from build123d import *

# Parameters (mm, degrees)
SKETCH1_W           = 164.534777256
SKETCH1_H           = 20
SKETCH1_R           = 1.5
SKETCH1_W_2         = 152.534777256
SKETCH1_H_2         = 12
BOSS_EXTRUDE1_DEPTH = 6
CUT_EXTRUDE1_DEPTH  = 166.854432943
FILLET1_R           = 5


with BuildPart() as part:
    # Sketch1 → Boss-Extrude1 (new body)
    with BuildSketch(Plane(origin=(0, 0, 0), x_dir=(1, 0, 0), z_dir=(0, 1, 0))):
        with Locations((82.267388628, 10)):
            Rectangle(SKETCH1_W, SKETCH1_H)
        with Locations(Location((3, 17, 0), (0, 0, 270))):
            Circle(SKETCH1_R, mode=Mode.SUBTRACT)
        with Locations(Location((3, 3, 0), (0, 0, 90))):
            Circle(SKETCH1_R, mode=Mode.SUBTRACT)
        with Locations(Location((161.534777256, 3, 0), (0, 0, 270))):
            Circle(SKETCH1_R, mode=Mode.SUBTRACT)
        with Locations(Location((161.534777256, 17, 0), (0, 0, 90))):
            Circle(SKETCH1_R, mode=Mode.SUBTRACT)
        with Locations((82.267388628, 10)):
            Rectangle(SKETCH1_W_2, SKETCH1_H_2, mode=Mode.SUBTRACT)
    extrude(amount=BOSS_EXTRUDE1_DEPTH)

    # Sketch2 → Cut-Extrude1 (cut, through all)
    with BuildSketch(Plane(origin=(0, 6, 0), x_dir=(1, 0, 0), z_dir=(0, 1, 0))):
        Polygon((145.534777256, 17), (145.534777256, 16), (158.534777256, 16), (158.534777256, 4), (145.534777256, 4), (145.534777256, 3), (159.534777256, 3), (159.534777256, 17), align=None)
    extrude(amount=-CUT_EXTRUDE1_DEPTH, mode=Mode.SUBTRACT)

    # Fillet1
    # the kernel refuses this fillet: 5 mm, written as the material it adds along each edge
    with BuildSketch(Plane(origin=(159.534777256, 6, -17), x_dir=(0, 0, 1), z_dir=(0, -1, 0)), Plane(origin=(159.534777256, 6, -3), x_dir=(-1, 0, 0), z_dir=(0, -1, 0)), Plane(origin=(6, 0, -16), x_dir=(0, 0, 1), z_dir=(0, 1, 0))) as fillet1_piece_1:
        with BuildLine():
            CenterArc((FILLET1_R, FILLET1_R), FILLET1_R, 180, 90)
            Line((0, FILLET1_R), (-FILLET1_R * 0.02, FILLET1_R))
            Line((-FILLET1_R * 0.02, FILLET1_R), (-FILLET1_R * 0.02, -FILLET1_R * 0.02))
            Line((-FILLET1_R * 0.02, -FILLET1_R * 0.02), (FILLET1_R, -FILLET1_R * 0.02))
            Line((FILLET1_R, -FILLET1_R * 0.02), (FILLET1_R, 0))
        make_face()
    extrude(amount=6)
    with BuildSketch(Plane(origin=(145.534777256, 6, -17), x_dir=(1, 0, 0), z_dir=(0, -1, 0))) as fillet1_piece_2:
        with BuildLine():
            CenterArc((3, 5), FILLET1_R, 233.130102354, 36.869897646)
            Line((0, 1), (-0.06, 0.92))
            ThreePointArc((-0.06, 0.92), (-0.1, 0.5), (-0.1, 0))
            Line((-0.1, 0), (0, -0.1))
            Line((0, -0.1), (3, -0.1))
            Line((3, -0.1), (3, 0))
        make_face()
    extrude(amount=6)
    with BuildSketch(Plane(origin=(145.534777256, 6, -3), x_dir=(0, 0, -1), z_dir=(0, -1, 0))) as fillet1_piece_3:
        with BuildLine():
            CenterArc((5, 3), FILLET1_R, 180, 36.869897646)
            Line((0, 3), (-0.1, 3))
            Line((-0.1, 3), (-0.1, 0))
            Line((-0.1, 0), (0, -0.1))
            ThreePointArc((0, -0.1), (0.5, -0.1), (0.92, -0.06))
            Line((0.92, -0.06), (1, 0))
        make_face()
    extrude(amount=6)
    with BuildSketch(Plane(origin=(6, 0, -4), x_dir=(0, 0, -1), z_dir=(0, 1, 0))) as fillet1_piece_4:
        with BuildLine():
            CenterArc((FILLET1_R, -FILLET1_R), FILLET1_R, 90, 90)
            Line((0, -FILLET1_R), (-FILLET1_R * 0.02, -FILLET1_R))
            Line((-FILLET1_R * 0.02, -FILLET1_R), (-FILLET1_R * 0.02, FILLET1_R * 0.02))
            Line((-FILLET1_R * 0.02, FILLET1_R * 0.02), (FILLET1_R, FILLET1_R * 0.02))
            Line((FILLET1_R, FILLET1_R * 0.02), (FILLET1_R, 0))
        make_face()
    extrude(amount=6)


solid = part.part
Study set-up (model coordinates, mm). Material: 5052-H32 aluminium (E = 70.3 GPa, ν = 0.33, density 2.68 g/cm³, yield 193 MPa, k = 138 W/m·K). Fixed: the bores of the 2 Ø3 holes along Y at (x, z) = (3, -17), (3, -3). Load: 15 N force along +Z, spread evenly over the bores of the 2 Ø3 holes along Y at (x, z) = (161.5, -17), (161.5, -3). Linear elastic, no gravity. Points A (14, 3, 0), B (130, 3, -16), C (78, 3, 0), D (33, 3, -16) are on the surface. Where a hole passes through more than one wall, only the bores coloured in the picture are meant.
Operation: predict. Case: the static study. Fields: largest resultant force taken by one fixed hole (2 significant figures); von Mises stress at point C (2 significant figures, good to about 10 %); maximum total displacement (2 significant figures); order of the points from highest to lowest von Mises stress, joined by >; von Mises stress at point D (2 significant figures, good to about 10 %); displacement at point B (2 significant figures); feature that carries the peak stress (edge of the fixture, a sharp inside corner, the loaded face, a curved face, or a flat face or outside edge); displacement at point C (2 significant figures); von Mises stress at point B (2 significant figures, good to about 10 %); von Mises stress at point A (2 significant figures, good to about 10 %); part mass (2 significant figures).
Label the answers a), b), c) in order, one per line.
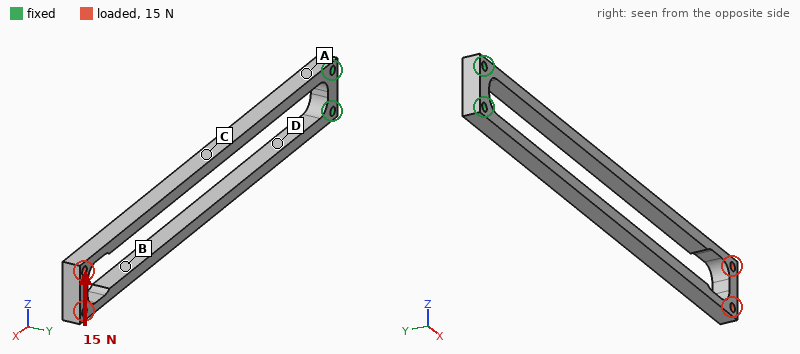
a) 120 N
b) 9.4 MPa
c) 1.3 mm
d) A > D > B > C
e) 25 MPa
f) 1.1 mm
g) a curved face
h) 0.53 mm
i) 20 MPa
j) 39 MPa
k) 23 g
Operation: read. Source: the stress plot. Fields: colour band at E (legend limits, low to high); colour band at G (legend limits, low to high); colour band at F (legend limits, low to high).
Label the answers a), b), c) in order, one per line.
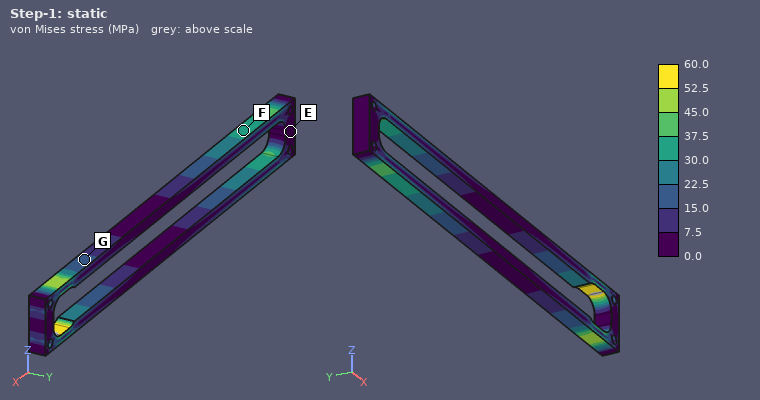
a) 0.0 to 7.5 MPa
b) 15.0 to 22.5 MPa
c) 30.0 to 37.5 MPa
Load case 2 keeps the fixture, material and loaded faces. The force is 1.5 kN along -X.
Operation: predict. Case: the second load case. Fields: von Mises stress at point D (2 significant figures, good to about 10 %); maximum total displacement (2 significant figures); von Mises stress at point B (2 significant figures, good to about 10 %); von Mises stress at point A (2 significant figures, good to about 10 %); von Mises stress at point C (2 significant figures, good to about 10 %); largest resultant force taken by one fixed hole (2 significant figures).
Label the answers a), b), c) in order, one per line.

a) 33 MPa
b) 82 µm
c) 28 MPa
d) 28 MPa
e) 32 MPa
f) 750 N
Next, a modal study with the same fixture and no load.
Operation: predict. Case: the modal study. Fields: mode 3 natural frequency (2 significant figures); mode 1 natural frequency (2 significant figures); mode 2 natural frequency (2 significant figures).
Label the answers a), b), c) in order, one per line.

a) 800 Hz
b) 190 Hz
c) 190 Hz
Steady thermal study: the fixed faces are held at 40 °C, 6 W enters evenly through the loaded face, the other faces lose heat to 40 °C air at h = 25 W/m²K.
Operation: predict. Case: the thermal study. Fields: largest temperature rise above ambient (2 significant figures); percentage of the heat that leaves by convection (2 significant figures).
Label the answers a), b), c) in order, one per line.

a) 67 K
b) 74 %
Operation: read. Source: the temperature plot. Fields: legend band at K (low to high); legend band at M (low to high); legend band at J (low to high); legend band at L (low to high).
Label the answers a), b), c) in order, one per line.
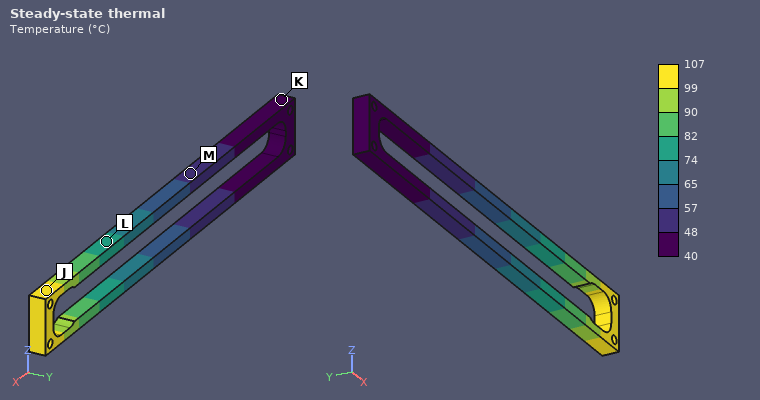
a) 40 to 48 °C
b) 48 to 57 °C
c) 99 to 107 °C
d) 74 to 82 °C
